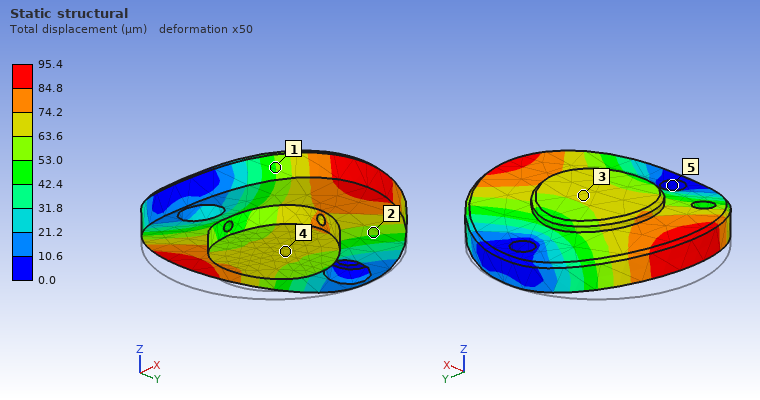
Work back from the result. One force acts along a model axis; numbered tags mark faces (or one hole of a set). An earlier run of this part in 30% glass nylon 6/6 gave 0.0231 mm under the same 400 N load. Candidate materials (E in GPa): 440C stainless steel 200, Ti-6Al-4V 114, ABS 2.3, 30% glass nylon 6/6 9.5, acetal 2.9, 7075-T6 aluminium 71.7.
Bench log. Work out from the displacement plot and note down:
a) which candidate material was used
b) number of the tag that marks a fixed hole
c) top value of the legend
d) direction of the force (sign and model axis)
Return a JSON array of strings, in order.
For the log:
["ABS", "5", "95.4 µm", "+Z"]
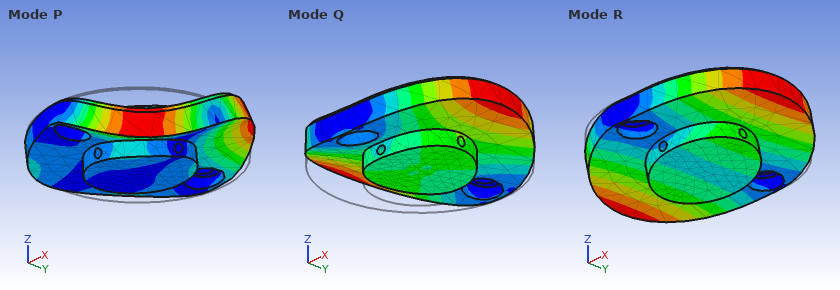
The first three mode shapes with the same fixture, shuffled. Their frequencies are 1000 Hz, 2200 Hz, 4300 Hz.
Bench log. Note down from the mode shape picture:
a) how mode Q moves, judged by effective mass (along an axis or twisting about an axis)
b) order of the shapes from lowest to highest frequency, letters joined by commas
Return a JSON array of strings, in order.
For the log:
["along Z", "R, Q, P"]
